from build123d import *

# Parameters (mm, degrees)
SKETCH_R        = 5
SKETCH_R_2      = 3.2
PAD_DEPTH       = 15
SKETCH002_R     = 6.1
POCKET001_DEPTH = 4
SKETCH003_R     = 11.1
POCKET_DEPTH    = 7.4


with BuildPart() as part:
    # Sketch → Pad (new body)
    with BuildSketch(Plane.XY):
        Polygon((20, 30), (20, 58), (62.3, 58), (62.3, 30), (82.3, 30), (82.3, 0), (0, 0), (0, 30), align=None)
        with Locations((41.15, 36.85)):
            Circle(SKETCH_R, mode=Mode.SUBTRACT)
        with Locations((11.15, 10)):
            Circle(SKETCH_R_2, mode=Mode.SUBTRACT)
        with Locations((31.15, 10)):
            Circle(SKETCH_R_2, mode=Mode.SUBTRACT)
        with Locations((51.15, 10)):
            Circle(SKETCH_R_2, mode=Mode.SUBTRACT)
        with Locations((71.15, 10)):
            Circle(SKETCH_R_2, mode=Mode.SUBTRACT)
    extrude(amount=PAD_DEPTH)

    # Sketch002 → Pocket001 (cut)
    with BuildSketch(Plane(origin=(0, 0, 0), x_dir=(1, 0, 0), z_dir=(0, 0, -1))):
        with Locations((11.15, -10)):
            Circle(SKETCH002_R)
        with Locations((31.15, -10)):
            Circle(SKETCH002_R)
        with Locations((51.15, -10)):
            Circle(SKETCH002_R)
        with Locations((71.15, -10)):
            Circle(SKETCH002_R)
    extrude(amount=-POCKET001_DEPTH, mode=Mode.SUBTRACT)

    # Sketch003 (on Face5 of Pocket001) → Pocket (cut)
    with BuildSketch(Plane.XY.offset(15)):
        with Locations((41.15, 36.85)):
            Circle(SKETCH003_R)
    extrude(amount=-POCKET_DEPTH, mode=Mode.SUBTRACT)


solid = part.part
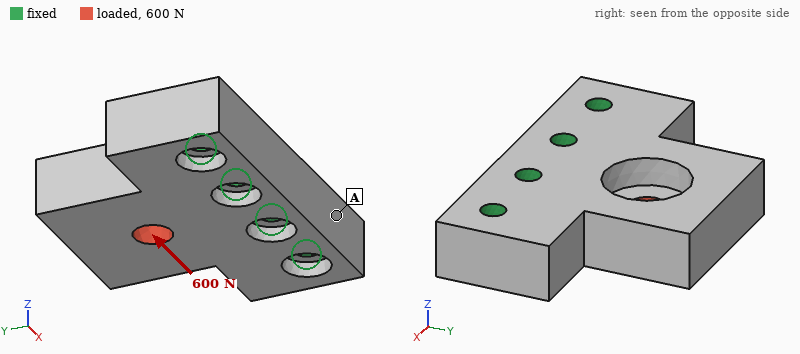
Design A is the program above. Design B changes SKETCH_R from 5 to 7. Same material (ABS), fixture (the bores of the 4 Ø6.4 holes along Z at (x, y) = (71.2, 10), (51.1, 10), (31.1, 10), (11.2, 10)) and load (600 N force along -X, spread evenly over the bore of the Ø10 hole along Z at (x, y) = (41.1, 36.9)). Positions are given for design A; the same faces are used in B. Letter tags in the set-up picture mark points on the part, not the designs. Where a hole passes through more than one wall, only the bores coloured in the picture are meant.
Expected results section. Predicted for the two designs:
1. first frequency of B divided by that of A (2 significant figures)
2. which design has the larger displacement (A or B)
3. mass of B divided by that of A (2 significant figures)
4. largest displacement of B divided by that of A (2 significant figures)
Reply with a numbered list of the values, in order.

1. 1.0
2. B
3. 0.99
4. 1.2
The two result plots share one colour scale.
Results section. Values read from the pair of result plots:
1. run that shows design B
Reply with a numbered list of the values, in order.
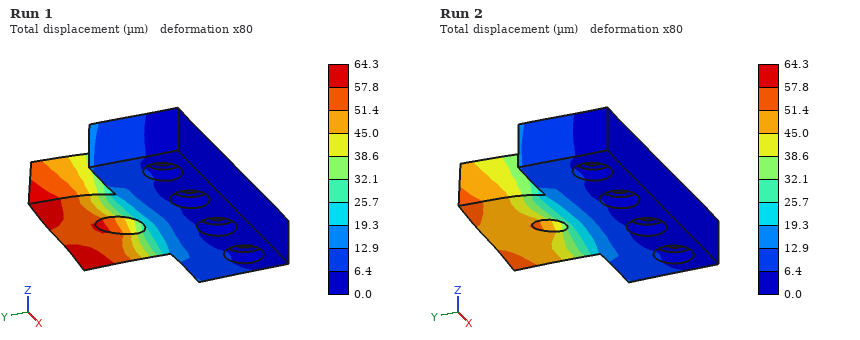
1. Run 1
